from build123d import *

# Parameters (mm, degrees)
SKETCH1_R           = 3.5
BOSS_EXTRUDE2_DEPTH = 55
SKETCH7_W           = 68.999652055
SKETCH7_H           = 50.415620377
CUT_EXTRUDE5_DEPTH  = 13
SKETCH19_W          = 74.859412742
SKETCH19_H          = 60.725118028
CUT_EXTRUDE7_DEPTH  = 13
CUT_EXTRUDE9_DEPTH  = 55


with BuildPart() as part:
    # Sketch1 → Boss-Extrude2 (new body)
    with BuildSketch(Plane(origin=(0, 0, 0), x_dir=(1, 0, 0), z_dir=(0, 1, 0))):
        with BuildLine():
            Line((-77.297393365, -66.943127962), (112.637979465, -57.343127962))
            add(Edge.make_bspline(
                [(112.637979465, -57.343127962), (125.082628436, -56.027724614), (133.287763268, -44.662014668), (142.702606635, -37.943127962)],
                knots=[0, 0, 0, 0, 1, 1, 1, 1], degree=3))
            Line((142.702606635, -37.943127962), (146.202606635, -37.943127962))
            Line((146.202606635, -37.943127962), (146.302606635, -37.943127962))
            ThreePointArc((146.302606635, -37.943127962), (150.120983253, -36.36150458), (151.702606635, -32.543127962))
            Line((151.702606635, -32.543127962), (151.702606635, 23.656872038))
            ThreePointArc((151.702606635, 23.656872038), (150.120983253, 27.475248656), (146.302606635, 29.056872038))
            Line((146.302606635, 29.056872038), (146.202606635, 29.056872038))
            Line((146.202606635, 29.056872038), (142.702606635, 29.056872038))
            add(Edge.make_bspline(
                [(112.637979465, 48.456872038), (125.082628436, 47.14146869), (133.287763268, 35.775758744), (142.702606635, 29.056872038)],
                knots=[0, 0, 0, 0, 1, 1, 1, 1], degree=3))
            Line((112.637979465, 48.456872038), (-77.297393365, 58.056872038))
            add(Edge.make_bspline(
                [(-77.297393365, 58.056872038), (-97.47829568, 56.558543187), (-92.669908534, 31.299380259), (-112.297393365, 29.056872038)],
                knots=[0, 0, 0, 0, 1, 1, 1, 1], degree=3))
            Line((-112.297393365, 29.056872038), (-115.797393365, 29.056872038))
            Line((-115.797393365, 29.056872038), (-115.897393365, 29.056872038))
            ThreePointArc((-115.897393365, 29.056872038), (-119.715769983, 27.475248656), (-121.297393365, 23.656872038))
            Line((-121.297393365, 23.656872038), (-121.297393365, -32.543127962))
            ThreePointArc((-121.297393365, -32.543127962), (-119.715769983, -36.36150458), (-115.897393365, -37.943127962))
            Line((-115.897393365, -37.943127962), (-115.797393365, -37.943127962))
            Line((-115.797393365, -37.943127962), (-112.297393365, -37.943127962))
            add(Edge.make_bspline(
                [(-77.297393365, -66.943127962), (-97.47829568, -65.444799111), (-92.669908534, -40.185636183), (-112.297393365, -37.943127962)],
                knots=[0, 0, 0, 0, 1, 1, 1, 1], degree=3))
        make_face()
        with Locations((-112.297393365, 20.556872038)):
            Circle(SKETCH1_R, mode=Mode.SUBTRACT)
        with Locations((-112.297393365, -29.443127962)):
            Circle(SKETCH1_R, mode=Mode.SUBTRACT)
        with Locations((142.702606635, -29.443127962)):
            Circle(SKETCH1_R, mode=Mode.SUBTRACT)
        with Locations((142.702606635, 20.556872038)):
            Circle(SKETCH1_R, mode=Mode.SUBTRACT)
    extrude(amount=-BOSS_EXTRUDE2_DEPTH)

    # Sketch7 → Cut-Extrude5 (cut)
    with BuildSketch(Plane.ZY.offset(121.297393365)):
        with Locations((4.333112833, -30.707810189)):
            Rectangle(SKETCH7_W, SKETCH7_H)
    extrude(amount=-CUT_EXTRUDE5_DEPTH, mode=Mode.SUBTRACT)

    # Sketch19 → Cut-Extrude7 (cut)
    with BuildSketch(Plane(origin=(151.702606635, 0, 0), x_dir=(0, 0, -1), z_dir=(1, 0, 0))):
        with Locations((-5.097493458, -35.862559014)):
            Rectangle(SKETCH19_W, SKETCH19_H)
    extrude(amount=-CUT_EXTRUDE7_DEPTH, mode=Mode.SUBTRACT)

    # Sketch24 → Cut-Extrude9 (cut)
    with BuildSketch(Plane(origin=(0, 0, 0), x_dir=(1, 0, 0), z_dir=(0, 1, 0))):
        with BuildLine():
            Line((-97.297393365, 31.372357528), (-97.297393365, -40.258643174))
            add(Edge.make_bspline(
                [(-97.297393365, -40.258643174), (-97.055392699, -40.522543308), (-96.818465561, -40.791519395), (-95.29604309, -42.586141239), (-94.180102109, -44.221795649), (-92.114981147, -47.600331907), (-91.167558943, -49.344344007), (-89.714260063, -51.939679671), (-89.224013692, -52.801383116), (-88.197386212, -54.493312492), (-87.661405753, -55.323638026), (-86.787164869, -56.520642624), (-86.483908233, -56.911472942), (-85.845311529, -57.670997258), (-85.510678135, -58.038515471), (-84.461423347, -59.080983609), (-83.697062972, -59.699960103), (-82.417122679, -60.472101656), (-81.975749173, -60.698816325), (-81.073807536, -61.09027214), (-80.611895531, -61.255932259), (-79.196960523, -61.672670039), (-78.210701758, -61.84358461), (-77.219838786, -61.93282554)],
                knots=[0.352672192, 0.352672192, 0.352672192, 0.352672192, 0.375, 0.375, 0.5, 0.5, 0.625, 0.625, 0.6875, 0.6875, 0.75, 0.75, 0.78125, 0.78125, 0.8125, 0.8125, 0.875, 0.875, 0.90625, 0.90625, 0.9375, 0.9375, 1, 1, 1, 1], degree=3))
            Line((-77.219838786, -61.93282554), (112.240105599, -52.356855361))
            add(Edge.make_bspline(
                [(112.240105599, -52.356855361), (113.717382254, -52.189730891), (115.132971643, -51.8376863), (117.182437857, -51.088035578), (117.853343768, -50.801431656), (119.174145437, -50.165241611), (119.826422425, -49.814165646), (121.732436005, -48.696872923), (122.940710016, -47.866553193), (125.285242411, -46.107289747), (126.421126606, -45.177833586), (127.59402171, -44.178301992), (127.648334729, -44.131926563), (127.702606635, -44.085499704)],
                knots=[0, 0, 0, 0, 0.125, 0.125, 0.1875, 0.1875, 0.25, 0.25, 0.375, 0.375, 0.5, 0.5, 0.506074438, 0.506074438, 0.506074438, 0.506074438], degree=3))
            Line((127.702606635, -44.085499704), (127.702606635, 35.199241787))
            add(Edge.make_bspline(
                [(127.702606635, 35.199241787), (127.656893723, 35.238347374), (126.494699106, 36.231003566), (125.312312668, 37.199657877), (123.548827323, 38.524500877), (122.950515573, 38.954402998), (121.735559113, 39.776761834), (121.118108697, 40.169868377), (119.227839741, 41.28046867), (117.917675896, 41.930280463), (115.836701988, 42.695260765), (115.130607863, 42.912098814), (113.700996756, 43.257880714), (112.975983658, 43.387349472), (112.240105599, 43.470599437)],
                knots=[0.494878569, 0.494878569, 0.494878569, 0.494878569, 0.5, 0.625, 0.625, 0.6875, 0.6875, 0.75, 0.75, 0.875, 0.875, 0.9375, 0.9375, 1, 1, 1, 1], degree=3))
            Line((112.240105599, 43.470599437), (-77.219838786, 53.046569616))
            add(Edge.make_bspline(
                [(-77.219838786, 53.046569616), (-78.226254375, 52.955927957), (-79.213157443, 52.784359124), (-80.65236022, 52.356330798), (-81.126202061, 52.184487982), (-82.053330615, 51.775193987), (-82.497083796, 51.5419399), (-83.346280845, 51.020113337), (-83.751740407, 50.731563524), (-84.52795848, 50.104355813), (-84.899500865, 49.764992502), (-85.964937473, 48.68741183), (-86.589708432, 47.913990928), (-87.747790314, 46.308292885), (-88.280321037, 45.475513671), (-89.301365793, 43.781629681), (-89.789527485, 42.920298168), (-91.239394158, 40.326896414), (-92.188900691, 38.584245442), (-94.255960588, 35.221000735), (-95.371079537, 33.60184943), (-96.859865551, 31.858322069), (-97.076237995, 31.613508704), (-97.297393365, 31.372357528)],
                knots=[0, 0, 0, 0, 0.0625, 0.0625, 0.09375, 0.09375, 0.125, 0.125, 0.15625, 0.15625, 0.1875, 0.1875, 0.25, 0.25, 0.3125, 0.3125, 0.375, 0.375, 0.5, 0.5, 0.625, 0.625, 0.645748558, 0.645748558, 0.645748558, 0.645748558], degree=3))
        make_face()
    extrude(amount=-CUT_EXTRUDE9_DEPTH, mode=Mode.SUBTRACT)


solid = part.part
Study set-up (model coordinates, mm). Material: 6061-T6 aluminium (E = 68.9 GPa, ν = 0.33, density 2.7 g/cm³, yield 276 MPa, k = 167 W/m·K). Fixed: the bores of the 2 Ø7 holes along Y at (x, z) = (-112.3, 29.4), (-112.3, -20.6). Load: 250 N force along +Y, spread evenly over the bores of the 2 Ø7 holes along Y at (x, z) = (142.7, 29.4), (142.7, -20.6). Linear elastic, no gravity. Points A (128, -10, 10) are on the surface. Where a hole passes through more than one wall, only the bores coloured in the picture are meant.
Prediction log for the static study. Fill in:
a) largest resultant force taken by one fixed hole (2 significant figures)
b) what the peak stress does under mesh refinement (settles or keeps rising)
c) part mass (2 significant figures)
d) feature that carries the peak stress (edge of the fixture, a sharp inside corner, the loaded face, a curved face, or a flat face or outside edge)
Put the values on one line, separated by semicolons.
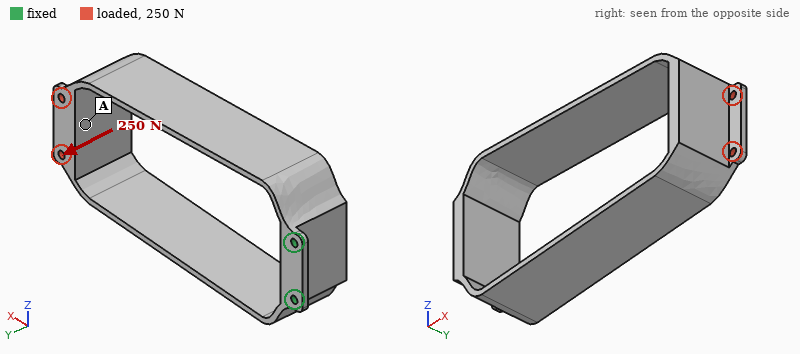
750 N; keeps rising; 640 g; edge of the fixture
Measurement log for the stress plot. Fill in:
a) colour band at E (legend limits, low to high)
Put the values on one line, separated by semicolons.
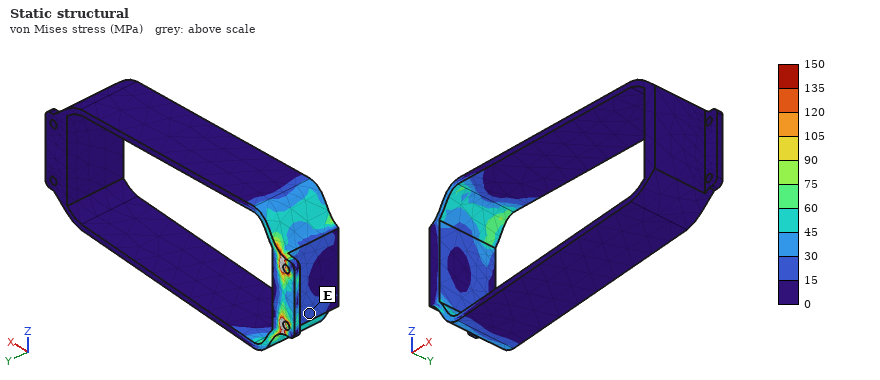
15 to 30 MPa
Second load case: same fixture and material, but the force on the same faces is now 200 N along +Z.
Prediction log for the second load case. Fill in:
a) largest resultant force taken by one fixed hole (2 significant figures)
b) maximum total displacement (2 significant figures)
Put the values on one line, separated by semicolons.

910 N; 3.0 mm
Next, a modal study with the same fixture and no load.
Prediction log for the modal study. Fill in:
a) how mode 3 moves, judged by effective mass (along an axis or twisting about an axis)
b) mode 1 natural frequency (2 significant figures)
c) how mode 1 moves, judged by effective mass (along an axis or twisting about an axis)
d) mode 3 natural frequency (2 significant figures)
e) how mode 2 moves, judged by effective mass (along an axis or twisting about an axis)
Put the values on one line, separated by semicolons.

twisting about X; 79 Hz; along Z; 380 Hz; along Y
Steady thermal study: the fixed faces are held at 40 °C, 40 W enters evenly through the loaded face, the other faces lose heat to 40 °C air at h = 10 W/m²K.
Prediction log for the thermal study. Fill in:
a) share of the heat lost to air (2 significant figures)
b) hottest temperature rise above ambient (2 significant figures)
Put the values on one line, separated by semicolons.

63 %; 76 K
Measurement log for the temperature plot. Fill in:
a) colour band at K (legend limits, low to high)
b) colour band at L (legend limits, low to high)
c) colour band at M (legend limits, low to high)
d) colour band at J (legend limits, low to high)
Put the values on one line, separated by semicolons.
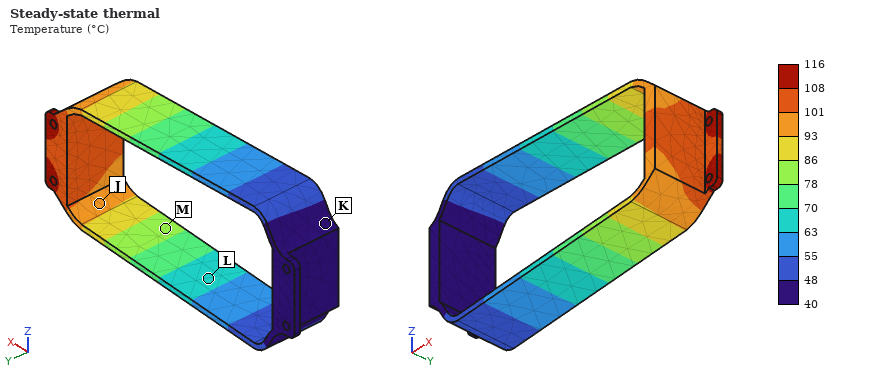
40 to 48 °C; 63 to 70 °C; 78 to 86 °C; 93 to 101 °C
